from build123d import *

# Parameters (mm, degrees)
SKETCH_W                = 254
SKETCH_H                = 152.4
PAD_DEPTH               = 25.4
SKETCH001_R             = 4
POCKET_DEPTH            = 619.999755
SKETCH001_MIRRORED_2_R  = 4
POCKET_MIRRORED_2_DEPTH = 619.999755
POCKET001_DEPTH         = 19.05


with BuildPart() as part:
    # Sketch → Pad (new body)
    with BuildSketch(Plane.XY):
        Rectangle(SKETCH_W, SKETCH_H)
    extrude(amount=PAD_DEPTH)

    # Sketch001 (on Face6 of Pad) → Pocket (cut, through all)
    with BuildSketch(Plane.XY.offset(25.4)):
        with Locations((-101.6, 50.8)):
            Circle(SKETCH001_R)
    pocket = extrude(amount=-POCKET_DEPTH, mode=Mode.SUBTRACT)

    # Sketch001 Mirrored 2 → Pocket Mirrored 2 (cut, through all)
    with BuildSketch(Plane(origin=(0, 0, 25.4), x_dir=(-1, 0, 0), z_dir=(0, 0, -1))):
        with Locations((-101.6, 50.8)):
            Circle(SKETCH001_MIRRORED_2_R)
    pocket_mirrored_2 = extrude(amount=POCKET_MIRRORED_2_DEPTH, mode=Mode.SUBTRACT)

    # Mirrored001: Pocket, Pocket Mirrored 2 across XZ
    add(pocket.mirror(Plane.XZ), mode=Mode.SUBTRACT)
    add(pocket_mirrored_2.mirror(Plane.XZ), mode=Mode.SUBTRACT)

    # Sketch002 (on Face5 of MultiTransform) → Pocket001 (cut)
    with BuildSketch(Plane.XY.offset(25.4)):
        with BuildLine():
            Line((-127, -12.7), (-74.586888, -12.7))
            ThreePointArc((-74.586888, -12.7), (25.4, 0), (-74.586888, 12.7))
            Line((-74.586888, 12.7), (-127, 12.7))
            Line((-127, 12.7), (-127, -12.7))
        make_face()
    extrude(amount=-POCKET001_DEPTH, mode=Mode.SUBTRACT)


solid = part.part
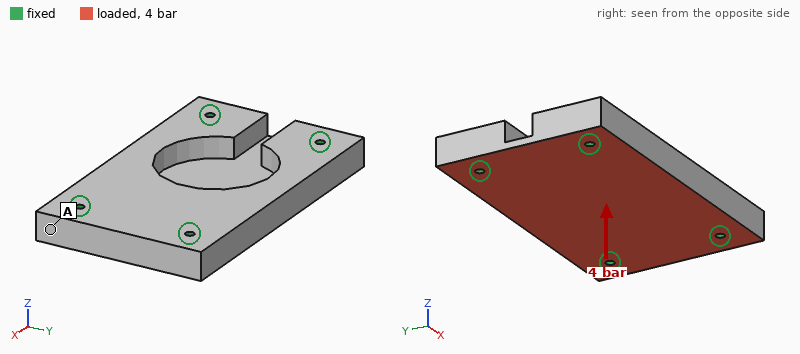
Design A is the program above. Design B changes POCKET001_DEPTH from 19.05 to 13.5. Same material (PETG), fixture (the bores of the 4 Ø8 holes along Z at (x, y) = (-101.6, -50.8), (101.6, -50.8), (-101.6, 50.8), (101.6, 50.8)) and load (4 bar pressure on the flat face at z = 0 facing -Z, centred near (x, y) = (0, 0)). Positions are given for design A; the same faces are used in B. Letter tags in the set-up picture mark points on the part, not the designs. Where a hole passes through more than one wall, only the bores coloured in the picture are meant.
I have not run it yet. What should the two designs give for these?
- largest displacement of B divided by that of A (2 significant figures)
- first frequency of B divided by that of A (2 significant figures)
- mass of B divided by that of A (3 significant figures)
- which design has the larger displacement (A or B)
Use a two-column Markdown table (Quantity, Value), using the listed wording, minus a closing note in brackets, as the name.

| Quantity | Value |
|---|---|
| largest displacement of B divided by that of A | 0.67 |
| first frequency of B divided by that of A | 0.97 |
| mass of B divided by that of A | 1.07 |
| which design has the larger displacement | A |
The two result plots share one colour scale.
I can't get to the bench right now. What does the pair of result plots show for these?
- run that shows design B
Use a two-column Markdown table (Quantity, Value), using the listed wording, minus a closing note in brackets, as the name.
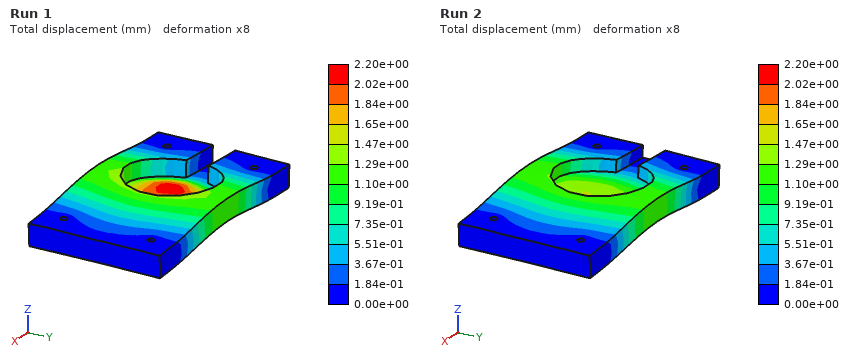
| Quantity | Value |
|---|---|
| run that shows design B | Run 2 |
